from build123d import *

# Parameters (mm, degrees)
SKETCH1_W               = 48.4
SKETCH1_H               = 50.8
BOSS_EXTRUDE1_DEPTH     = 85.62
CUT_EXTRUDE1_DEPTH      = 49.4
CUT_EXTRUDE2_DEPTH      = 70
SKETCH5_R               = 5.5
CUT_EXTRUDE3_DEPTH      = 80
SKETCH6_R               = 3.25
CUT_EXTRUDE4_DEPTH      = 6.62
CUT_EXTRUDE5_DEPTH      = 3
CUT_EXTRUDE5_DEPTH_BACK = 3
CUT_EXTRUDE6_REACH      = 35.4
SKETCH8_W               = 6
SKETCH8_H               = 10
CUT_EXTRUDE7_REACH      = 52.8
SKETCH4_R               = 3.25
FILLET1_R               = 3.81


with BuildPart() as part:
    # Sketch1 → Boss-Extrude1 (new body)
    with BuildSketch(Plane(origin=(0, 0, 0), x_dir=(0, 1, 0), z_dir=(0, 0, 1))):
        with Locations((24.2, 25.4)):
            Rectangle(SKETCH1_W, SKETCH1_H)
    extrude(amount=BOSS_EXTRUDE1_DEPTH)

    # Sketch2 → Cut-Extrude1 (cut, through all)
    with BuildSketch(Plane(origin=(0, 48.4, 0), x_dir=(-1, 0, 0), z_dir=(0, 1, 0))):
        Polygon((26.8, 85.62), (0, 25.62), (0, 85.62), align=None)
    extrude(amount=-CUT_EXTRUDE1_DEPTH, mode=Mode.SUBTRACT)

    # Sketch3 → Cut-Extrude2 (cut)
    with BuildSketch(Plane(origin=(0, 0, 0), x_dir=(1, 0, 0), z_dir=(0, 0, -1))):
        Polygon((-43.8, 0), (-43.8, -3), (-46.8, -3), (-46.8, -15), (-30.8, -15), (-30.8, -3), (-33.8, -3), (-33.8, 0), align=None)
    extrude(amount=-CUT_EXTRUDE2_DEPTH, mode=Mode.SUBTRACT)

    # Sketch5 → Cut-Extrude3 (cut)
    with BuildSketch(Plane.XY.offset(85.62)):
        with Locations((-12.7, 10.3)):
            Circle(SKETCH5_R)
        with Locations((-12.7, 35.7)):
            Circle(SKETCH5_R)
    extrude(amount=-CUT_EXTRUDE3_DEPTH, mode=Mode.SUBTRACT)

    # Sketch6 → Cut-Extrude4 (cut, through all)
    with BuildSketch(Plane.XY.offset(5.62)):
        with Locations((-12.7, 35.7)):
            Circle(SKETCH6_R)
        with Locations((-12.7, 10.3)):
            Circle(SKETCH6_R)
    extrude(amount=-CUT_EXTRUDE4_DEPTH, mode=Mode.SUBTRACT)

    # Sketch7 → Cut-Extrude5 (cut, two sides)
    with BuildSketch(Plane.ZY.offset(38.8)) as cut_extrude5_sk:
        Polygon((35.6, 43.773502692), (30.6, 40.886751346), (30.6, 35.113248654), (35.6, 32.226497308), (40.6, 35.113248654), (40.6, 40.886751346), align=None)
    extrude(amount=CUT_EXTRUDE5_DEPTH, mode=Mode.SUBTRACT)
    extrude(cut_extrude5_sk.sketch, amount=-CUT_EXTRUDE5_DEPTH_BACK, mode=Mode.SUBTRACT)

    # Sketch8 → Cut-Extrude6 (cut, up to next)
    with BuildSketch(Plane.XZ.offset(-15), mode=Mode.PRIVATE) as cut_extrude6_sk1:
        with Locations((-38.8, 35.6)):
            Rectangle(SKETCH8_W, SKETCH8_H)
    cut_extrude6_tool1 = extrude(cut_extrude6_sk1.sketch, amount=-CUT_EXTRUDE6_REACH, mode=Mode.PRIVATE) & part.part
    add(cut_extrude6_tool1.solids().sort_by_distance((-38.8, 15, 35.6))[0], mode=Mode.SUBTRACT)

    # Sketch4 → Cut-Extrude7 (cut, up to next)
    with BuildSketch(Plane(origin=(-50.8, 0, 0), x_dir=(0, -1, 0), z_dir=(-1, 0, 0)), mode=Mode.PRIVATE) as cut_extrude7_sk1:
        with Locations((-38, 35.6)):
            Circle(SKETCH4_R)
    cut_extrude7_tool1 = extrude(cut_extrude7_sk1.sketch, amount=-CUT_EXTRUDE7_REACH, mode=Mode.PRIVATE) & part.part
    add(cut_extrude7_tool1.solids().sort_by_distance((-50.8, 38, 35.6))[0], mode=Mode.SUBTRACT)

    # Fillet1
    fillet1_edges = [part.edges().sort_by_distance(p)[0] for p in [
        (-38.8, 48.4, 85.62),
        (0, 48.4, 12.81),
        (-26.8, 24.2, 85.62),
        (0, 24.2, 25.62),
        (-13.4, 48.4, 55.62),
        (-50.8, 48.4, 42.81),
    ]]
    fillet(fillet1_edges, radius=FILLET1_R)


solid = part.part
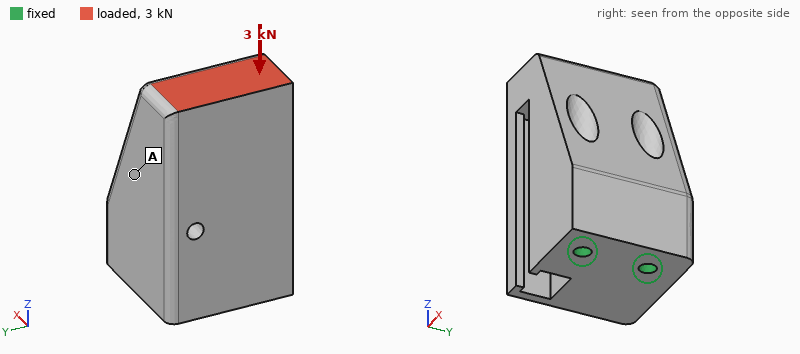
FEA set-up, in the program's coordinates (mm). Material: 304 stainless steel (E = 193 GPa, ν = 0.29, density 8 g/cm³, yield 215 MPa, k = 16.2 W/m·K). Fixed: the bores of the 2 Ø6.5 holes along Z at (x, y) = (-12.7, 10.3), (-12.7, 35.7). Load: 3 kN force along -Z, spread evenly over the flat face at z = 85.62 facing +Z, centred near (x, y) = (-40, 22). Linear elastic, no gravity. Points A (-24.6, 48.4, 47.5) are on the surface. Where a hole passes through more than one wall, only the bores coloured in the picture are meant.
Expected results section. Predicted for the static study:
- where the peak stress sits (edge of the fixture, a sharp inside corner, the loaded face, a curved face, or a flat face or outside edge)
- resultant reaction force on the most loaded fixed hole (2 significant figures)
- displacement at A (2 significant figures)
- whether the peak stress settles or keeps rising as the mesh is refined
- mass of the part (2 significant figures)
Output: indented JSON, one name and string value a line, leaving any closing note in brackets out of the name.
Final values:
{
  "where the peak stress sits": "edge of the fixture",
  "resultant reaction force on the most loaded fixed hole": "1.6 kN",
  "displacement at A": "48 µm",
  "whether the peak stress settles or keeps rising as the mesh is refined": "keeps rising",
  "mass of the part": "1.2 kg"
}
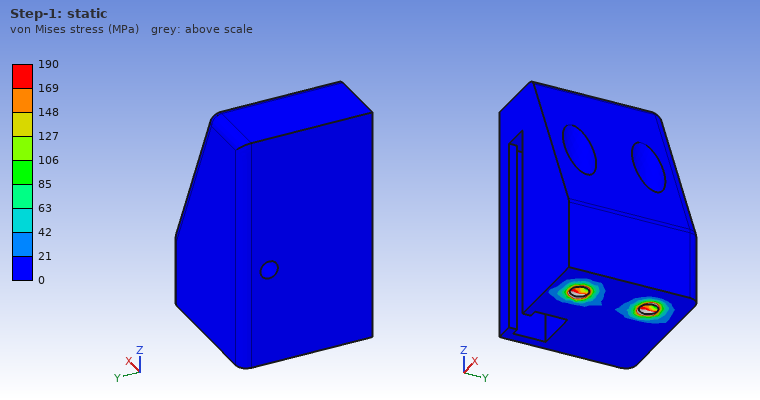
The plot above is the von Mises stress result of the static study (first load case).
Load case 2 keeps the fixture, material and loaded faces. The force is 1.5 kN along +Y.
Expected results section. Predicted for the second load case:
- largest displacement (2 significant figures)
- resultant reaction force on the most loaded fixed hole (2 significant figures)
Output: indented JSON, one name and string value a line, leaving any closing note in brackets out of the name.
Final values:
{
  "largest displacement": "26 µm",
  "resultant reaction force on the most loaded fixed hole": "4.6 kN"
}
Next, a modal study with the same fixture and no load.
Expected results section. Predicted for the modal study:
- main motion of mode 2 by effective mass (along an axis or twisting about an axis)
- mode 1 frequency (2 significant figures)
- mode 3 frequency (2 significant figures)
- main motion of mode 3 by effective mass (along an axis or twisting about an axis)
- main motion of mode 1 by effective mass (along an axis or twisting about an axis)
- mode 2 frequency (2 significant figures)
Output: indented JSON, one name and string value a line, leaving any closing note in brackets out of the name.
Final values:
{
  "main motion of mode 2 by effective mass": "along Y",
  "mode 1 frequency": "860 Hz",
  "mode 3 frequency": "5500 Hz",
  "main motion of mode 3 by effective mass": "twisting about Z",
  "main motion of mode 1 by effective mass": "along X",
  "mode 2 frequency": "2200 Hz"
}
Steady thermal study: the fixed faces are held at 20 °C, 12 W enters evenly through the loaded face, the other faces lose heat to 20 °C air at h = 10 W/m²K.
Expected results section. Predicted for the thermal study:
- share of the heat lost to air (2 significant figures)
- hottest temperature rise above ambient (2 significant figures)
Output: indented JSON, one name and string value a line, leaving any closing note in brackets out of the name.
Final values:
{
  "share of the heat lost to air": "38 %",
  "hottest temperature rise above ambient": "46 K"
}
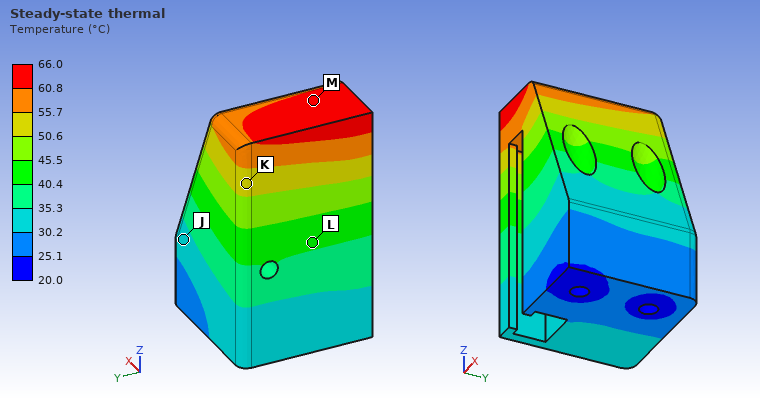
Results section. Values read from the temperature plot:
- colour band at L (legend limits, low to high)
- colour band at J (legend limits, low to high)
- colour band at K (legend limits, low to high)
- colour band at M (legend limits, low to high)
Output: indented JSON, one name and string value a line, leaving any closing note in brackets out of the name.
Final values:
{
  "colour band at L": "40.4 to 45.5 °C",
  "colour band at J": "30.2 to 35.3 °C",
  "colour band at K": "50.6 to 55.7 °C",
  "colour band at M": "60.8 to 66.0 °C"
}
